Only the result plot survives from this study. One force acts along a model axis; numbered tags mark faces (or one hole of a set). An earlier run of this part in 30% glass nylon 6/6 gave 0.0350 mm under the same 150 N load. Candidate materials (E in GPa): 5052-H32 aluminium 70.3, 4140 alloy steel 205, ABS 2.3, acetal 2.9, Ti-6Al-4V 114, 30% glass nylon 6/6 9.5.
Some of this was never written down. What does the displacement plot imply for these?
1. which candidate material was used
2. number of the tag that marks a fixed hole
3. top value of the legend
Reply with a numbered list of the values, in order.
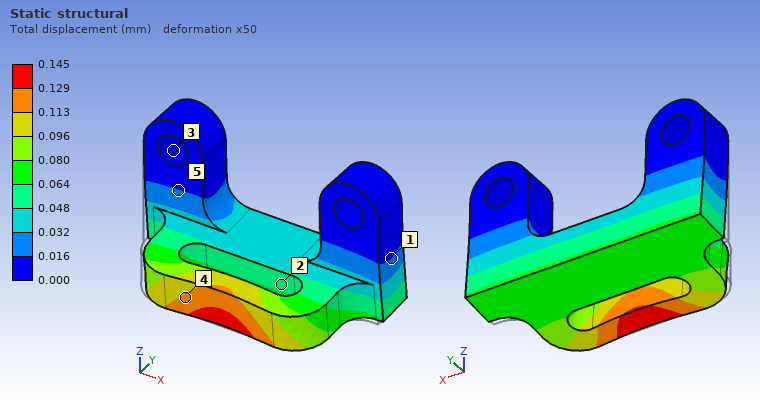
1. ABS
2. 3
3. 0.145 mm
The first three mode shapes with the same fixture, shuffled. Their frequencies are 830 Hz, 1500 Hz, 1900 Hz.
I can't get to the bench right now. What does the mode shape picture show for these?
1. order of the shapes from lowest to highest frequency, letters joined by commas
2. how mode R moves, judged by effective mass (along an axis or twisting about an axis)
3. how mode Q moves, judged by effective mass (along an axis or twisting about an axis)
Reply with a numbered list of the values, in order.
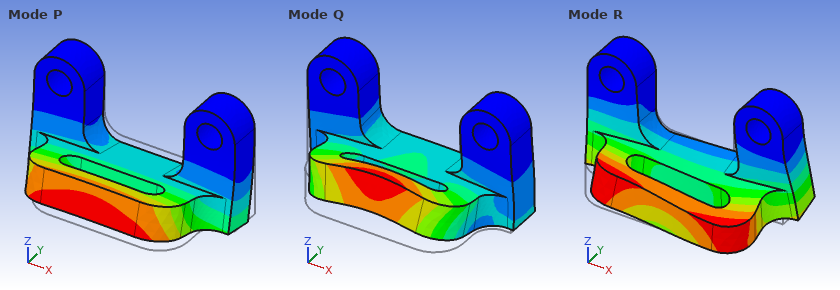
1. P, R, Q
2. along X
3. along Y
